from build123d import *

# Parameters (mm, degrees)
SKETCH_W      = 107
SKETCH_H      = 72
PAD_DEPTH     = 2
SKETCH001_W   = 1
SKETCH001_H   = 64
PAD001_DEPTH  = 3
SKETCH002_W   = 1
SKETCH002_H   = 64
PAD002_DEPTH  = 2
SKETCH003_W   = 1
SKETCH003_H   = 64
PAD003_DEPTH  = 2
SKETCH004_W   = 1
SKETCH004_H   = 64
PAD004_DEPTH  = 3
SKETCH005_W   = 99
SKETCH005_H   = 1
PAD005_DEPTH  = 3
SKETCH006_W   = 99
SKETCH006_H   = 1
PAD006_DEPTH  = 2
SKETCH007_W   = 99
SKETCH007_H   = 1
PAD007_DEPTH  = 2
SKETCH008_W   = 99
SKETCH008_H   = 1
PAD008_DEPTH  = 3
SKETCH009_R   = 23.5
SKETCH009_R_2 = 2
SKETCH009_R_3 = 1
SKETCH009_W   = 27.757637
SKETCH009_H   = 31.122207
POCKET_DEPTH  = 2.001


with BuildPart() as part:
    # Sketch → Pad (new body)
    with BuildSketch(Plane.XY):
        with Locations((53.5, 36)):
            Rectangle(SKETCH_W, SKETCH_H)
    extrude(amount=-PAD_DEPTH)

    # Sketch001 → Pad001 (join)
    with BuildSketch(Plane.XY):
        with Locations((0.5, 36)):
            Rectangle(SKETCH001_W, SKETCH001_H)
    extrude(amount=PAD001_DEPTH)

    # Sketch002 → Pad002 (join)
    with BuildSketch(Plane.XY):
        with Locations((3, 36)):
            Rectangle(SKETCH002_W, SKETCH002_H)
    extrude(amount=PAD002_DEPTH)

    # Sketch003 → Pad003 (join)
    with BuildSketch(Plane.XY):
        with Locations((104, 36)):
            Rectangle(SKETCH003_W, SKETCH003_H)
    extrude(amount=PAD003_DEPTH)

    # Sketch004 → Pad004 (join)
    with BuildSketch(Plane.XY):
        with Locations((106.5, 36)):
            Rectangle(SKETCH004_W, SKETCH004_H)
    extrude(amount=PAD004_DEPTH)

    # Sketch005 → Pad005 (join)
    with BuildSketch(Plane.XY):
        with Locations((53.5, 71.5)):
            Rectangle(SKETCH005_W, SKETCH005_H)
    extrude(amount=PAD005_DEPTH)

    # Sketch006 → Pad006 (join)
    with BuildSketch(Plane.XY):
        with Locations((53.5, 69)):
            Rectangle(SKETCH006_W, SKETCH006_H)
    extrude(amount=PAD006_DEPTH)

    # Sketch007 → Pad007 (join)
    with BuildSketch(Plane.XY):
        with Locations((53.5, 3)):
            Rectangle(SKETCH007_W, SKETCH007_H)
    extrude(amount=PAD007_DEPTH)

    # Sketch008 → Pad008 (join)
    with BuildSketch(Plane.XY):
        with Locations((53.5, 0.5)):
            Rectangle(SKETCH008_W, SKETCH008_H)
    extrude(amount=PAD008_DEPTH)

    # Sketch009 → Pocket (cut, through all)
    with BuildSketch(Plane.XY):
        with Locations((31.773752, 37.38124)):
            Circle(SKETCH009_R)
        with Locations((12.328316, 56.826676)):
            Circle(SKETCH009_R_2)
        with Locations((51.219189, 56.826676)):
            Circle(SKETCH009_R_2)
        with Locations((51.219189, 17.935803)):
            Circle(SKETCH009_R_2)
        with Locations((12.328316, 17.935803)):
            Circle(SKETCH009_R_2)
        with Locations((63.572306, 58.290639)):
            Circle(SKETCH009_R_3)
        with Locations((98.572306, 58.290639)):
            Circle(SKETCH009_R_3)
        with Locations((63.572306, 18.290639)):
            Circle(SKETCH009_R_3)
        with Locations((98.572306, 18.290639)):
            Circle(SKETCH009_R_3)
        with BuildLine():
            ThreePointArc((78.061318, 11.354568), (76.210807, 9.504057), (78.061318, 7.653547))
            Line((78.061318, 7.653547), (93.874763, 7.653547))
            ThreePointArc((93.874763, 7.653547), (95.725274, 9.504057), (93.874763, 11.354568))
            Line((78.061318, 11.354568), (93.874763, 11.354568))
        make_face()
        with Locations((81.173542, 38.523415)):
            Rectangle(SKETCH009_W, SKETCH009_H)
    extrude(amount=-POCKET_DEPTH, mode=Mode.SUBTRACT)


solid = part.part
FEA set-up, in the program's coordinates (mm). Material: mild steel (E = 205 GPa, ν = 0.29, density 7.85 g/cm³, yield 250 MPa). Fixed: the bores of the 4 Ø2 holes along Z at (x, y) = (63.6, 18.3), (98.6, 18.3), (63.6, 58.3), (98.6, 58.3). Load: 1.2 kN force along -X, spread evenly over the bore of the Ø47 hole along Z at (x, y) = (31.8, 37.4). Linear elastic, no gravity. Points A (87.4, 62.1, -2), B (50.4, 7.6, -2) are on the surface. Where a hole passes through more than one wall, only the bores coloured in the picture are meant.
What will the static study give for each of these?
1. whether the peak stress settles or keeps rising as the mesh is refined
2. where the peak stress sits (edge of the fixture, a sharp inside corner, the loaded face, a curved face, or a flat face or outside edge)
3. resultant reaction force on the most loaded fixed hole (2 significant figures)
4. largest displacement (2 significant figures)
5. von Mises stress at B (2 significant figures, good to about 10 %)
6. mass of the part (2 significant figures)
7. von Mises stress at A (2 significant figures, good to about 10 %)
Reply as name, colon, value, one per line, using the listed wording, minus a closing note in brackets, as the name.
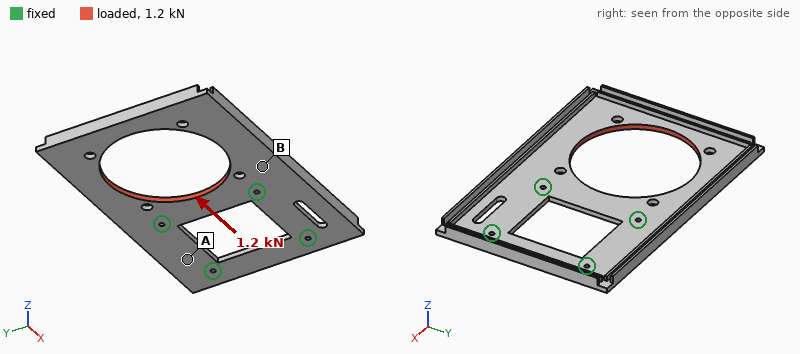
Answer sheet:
whether the peak stress settles or keeps rising as the mesh is refined: keeps rising
where the peak stress sits: edge of the fixture
resultant reaction force on the most loaded fixed hole: 460 N
largest displacement: 29 µm
von Mises stress at B: 15 MPa
mass of the part: 91 g
von Mises stress at A: 5.8 MPa
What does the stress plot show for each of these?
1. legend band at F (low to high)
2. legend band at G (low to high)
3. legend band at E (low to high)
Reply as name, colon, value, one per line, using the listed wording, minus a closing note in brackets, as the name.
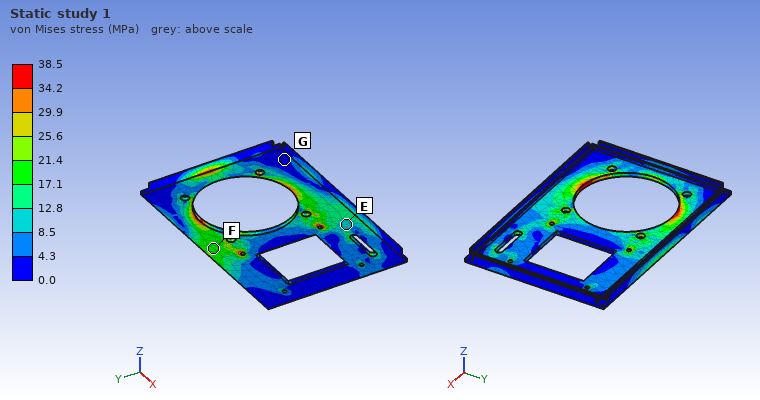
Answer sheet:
legend band at F: 17.1 to 21.4 MPa
legend band at G: 0.0 to 4.3 MPa
legend band at E: 8.5 to 12.8 MPa
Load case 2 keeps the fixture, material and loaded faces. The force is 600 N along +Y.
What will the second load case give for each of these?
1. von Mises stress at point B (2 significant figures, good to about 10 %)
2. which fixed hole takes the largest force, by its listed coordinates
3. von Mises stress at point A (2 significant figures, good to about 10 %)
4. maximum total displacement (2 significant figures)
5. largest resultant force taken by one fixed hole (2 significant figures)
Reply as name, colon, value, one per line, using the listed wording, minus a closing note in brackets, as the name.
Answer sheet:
von Mises stress at point B: 11 MPa
which fixed hole takes the largest force, by its listed coordinates: (63.6, 18.3)
von Mises stress at point A: 7.0 MPa
maximum total displacement: 40 µm
largest resultant force taken by one fixed hole: 450 N
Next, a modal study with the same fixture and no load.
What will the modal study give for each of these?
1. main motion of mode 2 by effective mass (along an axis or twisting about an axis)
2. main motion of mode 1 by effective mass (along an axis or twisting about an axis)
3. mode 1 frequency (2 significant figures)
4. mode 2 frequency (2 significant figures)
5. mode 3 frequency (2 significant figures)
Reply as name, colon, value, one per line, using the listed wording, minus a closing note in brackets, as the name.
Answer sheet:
main motion of mode 2 by effective mass: twisting about X
main motion of mode 1 by effective mass: along Z
mode 1 frequency: 440 Hz
mode 2 frequency: 750 Hz
mode 3 frequency: 2400 Hz
